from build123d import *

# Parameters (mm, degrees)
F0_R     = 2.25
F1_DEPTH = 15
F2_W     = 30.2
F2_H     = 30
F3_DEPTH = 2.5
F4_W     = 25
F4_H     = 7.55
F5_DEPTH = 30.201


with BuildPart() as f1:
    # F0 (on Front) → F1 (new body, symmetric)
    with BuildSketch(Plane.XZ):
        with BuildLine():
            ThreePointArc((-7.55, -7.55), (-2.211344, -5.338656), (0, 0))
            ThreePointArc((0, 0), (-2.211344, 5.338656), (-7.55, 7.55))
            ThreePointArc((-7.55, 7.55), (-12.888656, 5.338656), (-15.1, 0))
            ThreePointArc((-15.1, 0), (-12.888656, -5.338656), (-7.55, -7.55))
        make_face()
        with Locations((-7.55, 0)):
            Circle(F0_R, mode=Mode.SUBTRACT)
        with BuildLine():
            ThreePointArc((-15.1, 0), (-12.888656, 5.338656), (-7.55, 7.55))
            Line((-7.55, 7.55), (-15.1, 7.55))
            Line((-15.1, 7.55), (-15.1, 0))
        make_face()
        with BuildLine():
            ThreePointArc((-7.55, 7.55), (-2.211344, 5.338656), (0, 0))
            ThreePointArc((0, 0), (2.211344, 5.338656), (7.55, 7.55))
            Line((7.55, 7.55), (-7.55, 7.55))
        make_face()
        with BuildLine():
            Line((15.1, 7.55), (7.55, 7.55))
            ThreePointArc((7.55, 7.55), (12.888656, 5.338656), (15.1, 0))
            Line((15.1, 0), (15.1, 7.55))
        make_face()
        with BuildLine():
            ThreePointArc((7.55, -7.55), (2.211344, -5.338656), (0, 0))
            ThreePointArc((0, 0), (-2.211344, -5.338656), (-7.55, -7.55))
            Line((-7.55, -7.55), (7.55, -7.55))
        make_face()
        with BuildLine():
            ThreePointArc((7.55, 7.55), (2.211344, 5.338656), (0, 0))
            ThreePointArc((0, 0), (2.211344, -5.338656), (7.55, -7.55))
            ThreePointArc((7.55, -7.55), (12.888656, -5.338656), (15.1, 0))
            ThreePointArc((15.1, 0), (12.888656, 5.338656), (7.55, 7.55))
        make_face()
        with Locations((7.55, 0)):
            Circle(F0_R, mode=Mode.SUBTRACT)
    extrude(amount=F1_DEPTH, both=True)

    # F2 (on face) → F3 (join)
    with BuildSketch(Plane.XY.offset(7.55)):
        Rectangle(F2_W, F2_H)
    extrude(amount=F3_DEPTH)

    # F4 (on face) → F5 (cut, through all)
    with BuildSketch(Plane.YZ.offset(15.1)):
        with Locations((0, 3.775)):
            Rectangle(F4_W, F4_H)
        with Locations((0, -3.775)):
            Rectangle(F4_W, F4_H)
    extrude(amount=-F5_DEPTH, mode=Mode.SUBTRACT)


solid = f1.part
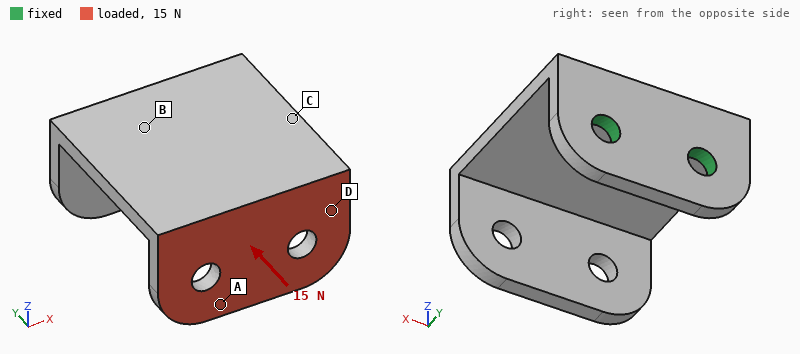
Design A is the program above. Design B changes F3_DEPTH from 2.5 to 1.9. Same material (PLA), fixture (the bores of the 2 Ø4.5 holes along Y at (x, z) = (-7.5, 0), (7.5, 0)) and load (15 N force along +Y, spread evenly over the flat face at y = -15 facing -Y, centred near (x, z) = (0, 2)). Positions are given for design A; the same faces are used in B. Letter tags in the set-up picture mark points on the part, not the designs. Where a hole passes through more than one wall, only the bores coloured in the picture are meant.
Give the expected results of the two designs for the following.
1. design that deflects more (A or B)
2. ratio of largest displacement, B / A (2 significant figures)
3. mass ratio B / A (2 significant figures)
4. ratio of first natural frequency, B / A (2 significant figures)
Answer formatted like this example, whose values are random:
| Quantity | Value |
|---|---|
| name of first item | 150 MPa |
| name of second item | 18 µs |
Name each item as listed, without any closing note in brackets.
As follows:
| Quantity | Value |
|---|---|
| design that deflects more | B |
| ratio of largest displacement, B / A | 2.0 |
| mass ratio B / A | 0.87 |
| ratio of first natural frequency, B / A | 0.81 |
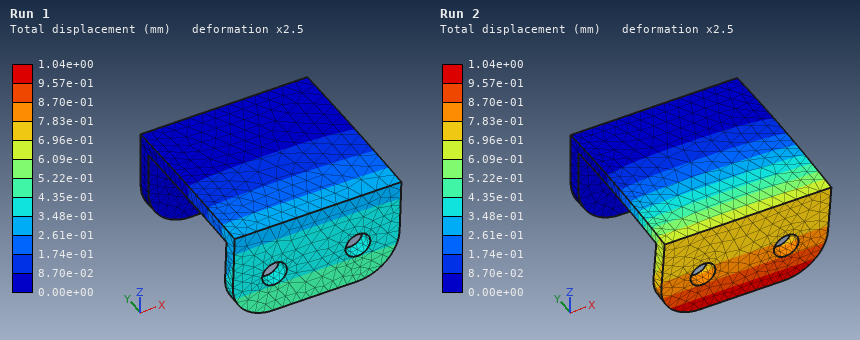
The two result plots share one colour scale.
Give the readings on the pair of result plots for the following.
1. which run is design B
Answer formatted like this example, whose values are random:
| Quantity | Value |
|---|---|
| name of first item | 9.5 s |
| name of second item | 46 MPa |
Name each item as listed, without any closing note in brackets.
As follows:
| Quantity | Value |
|---|---|
| which run is design B | Run 2 |
